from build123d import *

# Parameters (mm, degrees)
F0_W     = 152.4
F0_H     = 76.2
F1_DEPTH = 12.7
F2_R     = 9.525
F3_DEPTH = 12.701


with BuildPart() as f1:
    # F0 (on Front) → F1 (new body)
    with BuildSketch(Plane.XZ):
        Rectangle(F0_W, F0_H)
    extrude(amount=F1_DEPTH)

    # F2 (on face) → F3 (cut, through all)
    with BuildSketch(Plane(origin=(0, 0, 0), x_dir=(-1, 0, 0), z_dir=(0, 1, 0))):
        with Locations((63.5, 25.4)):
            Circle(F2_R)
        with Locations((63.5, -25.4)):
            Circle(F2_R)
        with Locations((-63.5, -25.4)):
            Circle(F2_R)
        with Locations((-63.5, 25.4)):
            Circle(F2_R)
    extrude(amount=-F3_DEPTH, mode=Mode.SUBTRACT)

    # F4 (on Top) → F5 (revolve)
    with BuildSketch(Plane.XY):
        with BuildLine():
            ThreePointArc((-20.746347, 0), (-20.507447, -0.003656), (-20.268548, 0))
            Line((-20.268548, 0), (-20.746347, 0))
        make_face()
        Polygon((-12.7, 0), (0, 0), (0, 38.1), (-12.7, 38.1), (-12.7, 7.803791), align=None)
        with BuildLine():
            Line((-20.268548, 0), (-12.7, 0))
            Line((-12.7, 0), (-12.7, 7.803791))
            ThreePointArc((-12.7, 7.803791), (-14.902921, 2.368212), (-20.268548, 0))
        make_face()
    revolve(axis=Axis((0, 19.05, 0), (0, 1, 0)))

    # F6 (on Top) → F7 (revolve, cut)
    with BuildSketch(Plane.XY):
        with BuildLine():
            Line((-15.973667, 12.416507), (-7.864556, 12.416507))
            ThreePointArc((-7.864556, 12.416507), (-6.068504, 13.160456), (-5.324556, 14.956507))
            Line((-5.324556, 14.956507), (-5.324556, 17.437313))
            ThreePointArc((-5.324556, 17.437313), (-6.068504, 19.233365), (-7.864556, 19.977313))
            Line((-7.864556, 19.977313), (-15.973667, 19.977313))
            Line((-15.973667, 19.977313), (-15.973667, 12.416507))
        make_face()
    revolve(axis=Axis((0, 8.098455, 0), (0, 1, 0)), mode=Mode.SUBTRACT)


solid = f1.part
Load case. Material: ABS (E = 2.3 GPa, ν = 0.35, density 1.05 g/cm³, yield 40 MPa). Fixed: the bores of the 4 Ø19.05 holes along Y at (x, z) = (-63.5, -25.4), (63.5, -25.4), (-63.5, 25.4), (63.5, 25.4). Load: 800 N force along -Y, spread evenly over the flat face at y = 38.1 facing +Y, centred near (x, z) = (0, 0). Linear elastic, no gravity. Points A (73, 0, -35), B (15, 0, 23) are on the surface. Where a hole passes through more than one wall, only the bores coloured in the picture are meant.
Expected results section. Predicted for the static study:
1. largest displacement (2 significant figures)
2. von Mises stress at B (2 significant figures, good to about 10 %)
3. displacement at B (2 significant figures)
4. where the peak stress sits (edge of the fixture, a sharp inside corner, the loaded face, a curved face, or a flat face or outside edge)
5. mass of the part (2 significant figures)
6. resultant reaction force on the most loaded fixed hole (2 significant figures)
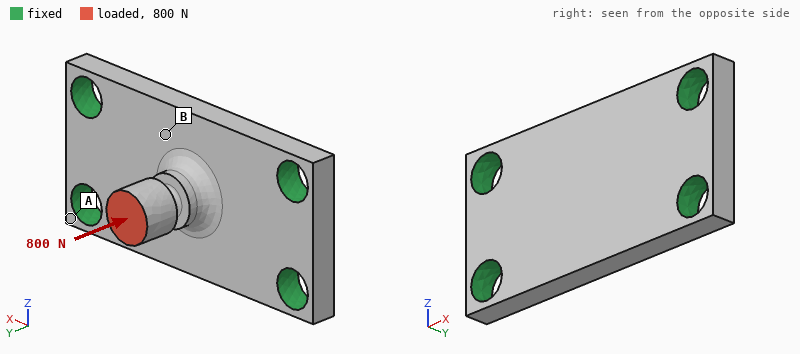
0.24 mm
2.2 MPa
0.15 mm
a curved face
160 g
210 N
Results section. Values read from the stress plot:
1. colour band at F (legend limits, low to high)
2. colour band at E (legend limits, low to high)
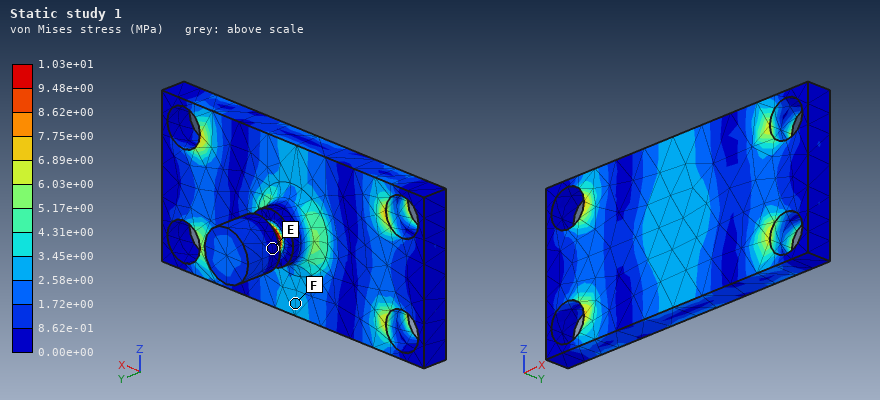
2.58e+00 to 3.45e+00 MPa
0.00e+00 to 8.62e-01 MPa
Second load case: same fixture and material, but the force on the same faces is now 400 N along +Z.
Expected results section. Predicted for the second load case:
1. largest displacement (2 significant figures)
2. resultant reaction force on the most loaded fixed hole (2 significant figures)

1.9 mm
220 N
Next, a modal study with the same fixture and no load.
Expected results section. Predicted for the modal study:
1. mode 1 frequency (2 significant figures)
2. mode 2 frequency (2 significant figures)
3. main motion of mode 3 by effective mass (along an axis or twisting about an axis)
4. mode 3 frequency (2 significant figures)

1100 Hz
1200 Hz
along Y
1300 Hz
